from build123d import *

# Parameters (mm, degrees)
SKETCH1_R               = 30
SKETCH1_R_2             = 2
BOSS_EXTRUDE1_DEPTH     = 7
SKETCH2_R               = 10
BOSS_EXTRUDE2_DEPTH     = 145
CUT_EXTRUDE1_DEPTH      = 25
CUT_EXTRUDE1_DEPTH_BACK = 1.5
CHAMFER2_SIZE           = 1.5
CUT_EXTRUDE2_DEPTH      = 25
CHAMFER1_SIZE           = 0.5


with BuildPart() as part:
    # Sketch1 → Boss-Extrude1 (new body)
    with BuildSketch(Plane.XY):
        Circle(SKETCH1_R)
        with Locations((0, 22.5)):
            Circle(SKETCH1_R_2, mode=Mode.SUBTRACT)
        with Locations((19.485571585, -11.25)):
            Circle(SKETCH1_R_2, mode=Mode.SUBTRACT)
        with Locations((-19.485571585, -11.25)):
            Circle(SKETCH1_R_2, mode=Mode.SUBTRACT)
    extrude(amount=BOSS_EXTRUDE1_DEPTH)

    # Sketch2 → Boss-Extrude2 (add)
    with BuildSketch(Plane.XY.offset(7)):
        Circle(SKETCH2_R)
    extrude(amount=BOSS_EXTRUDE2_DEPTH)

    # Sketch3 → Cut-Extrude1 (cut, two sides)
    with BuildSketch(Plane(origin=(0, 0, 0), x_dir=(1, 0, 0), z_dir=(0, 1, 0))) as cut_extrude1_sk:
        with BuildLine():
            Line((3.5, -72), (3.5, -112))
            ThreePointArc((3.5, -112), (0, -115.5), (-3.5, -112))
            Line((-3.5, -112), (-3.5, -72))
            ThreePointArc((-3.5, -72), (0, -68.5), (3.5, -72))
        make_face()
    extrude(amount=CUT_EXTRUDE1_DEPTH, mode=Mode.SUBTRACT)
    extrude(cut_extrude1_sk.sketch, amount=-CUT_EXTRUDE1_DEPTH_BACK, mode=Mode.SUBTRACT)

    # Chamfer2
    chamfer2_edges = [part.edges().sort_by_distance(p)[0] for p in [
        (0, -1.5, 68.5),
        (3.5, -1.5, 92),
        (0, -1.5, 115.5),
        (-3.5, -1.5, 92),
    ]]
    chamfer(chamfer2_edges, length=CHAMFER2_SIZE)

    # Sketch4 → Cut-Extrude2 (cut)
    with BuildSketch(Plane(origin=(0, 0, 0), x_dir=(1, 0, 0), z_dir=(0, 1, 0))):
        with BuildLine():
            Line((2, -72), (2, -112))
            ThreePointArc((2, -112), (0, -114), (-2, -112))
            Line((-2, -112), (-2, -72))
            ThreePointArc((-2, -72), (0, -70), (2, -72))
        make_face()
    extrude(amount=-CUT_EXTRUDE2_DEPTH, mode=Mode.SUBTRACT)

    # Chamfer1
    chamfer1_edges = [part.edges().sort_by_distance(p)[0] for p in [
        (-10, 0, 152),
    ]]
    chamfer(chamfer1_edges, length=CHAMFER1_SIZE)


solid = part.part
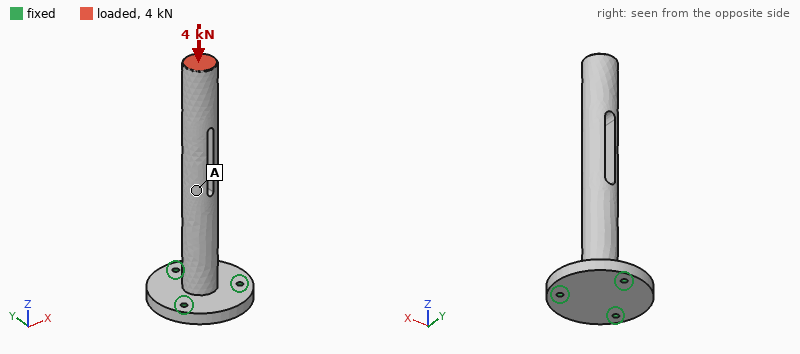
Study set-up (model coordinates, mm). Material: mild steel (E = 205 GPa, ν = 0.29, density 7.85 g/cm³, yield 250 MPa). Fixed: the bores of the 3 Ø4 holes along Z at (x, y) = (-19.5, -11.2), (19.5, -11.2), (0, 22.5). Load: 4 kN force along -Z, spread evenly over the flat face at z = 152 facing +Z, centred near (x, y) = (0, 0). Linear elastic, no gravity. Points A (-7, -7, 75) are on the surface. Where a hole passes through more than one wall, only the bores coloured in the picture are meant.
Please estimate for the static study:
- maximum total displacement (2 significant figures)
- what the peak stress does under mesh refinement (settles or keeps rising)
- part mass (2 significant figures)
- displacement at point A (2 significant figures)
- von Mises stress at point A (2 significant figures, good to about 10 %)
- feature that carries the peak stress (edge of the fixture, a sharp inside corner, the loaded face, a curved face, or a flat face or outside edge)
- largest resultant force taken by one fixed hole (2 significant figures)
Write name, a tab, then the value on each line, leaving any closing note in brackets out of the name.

maximum total displacement	21 µm
what the peak stress does under mesh refinement	keeps rising
part mass	470 g
displacement at point A	10 µm
von Mises stress at point A	15 MPa
feature that carries the peak stress	edge of the fixture
largest resultant force taken by one fixed hole	1.4 kN
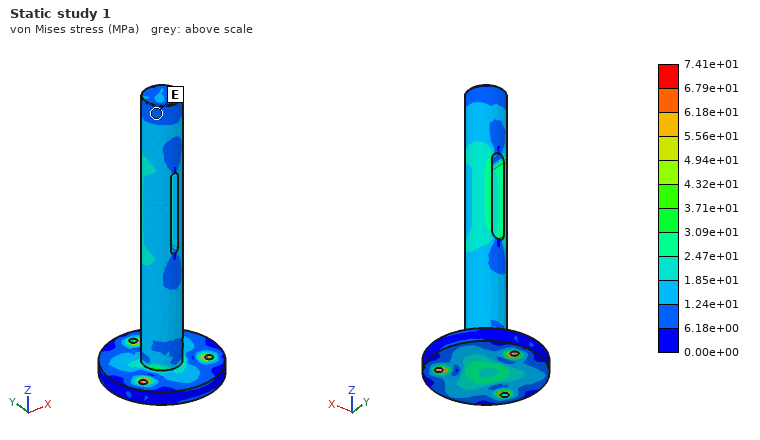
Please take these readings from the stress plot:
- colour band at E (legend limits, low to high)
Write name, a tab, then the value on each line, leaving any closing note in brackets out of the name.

colour band at E	6.18e+00 to 1.24e+01 MPa
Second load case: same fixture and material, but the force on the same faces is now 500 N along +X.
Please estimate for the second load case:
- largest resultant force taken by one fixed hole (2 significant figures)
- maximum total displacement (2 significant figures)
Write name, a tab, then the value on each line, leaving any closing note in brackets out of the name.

largest resultant force taken by one fixed hole	1.9 kN
maximum total displacement	0.46 mm
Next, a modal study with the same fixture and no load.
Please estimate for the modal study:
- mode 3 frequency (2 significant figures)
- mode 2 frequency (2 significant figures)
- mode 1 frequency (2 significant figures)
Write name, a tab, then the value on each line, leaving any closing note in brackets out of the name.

mode 3 frequency	3200 Hz
mode 2 frequency	570 Hz
mode 1 frequency	570 Hz
